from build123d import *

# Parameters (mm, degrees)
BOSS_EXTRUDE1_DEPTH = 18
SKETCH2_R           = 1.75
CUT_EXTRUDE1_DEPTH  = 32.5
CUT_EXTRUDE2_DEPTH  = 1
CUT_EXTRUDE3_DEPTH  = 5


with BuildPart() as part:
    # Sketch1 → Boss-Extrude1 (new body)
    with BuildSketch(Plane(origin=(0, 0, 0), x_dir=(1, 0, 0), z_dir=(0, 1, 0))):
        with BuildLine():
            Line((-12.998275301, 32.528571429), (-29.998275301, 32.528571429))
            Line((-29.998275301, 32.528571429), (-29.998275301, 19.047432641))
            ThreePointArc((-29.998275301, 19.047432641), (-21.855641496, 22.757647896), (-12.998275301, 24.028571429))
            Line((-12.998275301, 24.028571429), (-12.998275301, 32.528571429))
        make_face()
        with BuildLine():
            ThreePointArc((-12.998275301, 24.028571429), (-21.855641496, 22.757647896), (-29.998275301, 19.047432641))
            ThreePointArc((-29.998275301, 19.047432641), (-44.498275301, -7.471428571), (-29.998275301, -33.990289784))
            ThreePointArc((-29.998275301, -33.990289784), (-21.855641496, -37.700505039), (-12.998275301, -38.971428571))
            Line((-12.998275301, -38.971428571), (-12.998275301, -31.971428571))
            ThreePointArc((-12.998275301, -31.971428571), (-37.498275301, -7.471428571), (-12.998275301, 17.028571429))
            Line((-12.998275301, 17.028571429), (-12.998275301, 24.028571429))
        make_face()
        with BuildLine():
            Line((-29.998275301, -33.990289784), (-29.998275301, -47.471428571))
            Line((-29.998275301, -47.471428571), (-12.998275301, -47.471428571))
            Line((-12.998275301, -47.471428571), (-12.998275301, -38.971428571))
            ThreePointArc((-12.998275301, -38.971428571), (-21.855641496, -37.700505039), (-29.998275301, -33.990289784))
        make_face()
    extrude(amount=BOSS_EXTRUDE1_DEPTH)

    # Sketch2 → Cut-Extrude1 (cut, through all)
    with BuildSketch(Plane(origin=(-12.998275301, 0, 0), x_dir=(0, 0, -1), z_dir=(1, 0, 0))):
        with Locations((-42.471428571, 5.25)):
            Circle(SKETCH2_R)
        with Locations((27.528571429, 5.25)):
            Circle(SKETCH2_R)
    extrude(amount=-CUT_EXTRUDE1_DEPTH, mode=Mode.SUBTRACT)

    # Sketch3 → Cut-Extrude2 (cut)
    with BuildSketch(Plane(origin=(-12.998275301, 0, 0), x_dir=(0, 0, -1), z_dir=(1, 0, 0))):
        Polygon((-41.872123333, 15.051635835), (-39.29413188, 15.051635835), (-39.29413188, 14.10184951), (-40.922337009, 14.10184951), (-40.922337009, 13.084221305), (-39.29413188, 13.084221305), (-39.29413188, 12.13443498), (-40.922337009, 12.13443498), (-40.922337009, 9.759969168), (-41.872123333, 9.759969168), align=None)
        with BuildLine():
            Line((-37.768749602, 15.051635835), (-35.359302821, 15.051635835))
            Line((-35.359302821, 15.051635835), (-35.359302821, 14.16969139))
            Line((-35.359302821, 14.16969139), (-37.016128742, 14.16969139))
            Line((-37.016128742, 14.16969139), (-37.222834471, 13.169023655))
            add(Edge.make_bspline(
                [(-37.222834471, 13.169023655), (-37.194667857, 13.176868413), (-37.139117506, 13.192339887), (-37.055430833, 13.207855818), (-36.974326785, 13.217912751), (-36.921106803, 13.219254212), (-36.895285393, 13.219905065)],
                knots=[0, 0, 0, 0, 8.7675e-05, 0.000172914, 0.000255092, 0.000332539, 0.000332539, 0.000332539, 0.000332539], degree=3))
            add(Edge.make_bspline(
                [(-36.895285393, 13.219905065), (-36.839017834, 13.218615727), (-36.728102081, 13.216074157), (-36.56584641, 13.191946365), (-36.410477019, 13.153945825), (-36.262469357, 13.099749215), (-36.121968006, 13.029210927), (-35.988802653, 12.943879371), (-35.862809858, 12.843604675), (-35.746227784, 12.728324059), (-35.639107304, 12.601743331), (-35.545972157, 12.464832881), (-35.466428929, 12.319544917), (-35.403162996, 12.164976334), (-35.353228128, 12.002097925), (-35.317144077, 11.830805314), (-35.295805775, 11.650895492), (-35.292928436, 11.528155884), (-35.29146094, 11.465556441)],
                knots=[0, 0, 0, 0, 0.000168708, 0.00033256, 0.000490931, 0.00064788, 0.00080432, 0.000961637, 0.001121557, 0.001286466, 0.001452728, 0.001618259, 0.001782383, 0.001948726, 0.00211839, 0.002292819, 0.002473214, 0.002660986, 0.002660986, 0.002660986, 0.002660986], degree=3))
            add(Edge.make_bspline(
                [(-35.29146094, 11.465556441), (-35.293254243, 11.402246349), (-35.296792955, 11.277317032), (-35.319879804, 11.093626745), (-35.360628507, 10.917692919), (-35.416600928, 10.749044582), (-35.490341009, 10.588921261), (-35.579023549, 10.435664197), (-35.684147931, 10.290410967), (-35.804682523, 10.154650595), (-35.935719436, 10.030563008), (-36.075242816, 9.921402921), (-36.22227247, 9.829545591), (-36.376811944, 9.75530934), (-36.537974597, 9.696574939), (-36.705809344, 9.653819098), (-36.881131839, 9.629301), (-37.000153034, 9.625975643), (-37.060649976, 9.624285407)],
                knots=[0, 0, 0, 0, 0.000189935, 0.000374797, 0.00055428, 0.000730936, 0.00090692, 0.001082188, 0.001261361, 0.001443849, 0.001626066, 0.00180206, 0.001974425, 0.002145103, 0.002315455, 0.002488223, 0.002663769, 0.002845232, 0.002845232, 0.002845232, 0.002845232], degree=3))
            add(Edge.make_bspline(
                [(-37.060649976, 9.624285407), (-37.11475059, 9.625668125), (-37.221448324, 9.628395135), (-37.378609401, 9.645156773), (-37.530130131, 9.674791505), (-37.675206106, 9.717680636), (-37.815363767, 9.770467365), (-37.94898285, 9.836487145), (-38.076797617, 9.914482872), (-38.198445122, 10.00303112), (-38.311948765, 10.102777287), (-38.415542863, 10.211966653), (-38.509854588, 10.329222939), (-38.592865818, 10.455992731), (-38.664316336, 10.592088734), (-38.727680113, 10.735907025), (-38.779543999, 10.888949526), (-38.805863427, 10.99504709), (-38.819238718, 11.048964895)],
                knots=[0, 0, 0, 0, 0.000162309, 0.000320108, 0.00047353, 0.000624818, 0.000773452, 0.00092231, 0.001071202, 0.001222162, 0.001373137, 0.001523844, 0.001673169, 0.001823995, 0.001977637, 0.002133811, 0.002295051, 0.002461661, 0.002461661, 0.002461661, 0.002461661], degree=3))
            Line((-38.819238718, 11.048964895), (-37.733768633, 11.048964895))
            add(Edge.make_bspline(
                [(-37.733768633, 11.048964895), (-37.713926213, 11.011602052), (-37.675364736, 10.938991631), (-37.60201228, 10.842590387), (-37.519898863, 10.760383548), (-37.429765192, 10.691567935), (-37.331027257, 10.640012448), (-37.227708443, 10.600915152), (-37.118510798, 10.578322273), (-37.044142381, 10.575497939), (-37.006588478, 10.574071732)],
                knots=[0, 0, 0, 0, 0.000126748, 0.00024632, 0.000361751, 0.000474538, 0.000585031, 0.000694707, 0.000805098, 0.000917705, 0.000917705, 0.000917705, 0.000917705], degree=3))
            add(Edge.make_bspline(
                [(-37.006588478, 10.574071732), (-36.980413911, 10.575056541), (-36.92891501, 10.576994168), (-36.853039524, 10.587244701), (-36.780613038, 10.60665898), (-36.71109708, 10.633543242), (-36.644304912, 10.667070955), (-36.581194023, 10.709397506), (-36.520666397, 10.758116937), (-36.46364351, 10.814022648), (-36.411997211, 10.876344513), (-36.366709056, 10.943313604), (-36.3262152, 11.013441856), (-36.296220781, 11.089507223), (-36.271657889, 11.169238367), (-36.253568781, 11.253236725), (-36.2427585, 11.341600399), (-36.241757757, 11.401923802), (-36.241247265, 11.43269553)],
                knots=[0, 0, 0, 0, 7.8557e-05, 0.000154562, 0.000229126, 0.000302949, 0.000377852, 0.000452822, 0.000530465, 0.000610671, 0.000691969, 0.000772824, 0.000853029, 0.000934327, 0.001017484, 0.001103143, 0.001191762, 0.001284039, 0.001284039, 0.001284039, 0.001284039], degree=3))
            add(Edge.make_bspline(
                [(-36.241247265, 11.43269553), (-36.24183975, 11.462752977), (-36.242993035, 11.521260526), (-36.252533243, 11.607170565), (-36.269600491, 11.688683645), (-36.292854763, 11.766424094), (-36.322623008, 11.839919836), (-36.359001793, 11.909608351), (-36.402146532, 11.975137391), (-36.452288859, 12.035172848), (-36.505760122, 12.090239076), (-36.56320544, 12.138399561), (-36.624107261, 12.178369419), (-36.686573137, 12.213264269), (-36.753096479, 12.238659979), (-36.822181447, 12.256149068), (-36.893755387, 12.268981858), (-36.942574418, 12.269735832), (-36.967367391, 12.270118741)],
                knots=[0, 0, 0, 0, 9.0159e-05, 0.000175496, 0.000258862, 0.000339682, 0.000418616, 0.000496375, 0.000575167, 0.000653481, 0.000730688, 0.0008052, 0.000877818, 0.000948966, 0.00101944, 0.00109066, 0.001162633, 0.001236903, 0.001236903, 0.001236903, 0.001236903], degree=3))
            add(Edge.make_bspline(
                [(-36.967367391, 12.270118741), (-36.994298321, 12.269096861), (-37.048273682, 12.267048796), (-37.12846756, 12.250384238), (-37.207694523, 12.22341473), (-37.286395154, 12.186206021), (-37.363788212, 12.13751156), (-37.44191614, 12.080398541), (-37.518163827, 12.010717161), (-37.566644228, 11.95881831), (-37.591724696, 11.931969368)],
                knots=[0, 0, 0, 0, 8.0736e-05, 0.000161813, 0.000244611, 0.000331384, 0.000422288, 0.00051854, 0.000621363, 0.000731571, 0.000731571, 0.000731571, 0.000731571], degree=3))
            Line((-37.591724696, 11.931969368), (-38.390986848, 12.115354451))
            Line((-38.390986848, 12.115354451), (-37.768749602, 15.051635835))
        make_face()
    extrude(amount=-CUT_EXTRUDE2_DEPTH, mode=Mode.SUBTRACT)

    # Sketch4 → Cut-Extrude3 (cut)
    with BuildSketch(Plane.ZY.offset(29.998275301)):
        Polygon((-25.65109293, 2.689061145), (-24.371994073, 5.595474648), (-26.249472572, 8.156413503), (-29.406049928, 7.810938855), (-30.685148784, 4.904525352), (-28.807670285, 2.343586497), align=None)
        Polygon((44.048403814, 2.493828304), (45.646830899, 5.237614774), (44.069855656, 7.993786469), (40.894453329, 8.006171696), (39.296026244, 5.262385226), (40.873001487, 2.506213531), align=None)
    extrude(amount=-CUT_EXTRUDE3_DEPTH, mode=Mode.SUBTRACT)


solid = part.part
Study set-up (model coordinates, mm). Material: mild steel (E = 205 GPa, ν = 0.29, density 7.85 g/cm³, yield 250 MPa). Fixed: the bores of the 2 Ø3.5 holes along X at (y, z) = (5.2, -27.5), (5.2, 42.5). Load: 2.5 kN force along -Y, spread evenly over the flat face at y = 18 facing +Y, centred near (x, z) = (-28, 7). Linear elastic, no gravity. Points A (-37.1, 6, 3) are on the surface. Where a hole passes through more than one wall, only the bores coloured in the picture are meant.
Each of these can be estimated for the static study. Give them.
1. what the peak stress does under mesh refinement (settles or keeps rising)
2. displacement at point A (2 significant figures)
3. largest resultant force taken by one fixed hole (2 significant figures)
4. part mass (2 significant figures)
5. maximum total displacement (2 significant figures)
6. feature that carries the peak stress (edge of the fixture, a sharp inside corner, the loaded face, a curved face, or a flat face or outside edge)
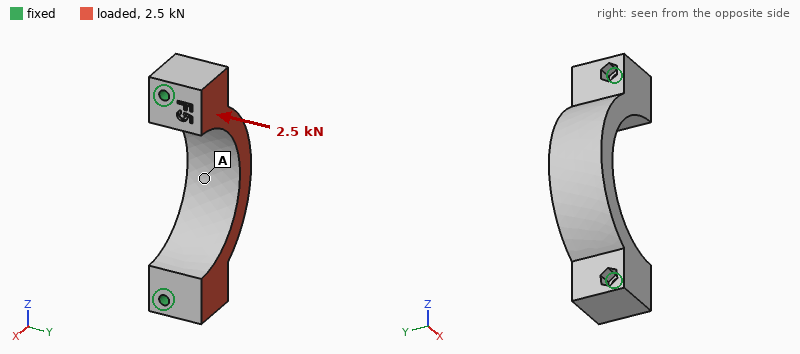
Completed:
keeps rising
11 µm
1.3 kN
130 g
16 µm
edge of the fixture
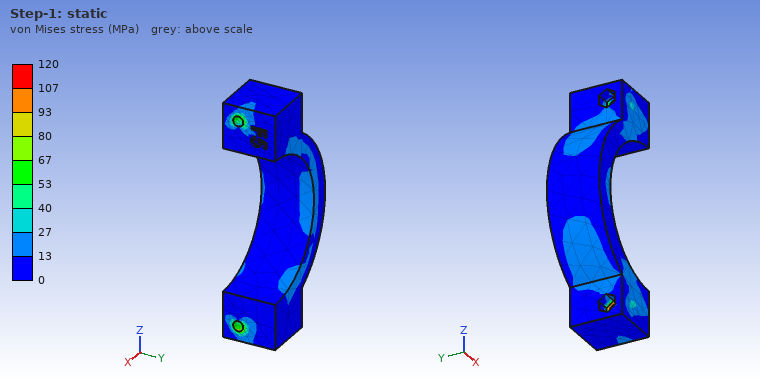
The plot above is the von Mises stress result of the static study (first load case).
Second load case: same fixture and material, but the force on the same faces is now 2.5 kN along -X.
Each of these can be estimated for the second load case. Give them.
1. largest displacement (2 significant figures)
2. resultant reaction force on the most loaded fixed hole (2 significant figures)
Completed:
14 µm
1.3 kN
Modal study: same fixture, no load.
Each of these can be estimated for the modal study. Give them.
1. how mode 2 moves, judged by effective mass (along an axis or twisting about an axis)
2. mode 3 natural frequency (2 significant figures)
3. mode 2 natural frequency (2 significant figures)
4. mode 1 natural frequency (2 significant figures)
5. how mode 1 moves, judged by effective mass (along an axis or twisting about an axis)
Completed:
along Z
18 kHz
13 kHz
6700 Hz
along Y
